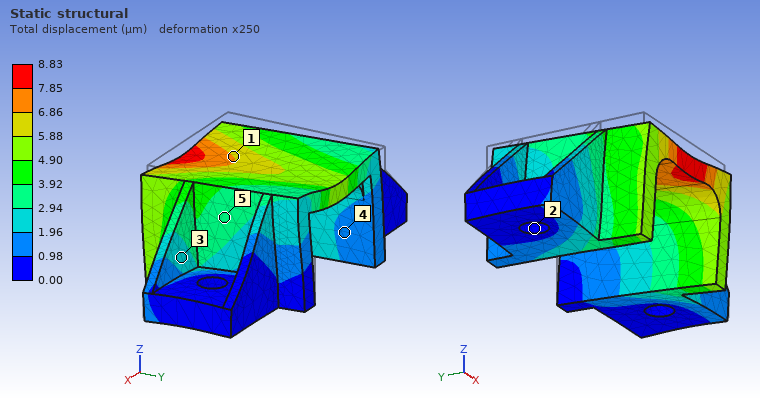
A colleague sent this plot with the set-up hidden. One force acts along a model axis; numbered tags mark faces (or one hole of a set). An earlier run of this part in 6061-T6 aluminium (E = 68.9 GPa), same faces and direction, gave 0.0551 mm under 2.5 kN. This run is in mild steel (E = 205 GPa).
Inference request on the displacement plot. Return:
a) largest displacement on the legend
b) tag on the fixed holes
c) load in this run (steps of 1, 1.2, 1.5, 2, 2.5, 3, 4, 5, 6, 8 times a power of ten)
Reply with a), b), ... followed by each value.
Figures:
a) 8.83 µm
b) 2
c) 1.2 kN
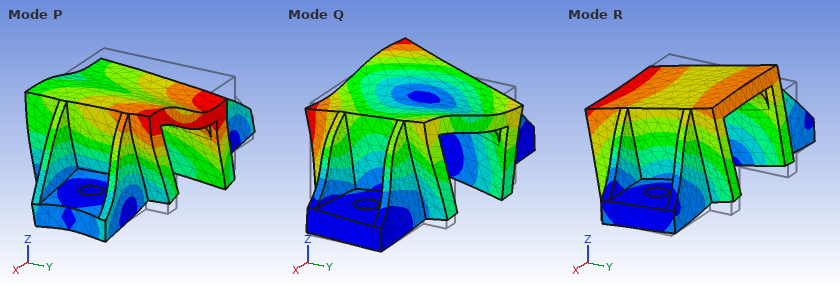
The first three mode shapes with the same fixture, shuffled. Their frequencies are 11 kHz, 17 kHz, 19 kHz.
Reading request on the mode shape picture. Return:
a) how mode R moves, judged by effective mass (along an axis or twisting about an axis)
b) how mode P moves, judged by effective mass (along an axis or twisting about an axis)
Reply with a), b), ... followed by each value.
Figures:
a) along Y
b) along X
